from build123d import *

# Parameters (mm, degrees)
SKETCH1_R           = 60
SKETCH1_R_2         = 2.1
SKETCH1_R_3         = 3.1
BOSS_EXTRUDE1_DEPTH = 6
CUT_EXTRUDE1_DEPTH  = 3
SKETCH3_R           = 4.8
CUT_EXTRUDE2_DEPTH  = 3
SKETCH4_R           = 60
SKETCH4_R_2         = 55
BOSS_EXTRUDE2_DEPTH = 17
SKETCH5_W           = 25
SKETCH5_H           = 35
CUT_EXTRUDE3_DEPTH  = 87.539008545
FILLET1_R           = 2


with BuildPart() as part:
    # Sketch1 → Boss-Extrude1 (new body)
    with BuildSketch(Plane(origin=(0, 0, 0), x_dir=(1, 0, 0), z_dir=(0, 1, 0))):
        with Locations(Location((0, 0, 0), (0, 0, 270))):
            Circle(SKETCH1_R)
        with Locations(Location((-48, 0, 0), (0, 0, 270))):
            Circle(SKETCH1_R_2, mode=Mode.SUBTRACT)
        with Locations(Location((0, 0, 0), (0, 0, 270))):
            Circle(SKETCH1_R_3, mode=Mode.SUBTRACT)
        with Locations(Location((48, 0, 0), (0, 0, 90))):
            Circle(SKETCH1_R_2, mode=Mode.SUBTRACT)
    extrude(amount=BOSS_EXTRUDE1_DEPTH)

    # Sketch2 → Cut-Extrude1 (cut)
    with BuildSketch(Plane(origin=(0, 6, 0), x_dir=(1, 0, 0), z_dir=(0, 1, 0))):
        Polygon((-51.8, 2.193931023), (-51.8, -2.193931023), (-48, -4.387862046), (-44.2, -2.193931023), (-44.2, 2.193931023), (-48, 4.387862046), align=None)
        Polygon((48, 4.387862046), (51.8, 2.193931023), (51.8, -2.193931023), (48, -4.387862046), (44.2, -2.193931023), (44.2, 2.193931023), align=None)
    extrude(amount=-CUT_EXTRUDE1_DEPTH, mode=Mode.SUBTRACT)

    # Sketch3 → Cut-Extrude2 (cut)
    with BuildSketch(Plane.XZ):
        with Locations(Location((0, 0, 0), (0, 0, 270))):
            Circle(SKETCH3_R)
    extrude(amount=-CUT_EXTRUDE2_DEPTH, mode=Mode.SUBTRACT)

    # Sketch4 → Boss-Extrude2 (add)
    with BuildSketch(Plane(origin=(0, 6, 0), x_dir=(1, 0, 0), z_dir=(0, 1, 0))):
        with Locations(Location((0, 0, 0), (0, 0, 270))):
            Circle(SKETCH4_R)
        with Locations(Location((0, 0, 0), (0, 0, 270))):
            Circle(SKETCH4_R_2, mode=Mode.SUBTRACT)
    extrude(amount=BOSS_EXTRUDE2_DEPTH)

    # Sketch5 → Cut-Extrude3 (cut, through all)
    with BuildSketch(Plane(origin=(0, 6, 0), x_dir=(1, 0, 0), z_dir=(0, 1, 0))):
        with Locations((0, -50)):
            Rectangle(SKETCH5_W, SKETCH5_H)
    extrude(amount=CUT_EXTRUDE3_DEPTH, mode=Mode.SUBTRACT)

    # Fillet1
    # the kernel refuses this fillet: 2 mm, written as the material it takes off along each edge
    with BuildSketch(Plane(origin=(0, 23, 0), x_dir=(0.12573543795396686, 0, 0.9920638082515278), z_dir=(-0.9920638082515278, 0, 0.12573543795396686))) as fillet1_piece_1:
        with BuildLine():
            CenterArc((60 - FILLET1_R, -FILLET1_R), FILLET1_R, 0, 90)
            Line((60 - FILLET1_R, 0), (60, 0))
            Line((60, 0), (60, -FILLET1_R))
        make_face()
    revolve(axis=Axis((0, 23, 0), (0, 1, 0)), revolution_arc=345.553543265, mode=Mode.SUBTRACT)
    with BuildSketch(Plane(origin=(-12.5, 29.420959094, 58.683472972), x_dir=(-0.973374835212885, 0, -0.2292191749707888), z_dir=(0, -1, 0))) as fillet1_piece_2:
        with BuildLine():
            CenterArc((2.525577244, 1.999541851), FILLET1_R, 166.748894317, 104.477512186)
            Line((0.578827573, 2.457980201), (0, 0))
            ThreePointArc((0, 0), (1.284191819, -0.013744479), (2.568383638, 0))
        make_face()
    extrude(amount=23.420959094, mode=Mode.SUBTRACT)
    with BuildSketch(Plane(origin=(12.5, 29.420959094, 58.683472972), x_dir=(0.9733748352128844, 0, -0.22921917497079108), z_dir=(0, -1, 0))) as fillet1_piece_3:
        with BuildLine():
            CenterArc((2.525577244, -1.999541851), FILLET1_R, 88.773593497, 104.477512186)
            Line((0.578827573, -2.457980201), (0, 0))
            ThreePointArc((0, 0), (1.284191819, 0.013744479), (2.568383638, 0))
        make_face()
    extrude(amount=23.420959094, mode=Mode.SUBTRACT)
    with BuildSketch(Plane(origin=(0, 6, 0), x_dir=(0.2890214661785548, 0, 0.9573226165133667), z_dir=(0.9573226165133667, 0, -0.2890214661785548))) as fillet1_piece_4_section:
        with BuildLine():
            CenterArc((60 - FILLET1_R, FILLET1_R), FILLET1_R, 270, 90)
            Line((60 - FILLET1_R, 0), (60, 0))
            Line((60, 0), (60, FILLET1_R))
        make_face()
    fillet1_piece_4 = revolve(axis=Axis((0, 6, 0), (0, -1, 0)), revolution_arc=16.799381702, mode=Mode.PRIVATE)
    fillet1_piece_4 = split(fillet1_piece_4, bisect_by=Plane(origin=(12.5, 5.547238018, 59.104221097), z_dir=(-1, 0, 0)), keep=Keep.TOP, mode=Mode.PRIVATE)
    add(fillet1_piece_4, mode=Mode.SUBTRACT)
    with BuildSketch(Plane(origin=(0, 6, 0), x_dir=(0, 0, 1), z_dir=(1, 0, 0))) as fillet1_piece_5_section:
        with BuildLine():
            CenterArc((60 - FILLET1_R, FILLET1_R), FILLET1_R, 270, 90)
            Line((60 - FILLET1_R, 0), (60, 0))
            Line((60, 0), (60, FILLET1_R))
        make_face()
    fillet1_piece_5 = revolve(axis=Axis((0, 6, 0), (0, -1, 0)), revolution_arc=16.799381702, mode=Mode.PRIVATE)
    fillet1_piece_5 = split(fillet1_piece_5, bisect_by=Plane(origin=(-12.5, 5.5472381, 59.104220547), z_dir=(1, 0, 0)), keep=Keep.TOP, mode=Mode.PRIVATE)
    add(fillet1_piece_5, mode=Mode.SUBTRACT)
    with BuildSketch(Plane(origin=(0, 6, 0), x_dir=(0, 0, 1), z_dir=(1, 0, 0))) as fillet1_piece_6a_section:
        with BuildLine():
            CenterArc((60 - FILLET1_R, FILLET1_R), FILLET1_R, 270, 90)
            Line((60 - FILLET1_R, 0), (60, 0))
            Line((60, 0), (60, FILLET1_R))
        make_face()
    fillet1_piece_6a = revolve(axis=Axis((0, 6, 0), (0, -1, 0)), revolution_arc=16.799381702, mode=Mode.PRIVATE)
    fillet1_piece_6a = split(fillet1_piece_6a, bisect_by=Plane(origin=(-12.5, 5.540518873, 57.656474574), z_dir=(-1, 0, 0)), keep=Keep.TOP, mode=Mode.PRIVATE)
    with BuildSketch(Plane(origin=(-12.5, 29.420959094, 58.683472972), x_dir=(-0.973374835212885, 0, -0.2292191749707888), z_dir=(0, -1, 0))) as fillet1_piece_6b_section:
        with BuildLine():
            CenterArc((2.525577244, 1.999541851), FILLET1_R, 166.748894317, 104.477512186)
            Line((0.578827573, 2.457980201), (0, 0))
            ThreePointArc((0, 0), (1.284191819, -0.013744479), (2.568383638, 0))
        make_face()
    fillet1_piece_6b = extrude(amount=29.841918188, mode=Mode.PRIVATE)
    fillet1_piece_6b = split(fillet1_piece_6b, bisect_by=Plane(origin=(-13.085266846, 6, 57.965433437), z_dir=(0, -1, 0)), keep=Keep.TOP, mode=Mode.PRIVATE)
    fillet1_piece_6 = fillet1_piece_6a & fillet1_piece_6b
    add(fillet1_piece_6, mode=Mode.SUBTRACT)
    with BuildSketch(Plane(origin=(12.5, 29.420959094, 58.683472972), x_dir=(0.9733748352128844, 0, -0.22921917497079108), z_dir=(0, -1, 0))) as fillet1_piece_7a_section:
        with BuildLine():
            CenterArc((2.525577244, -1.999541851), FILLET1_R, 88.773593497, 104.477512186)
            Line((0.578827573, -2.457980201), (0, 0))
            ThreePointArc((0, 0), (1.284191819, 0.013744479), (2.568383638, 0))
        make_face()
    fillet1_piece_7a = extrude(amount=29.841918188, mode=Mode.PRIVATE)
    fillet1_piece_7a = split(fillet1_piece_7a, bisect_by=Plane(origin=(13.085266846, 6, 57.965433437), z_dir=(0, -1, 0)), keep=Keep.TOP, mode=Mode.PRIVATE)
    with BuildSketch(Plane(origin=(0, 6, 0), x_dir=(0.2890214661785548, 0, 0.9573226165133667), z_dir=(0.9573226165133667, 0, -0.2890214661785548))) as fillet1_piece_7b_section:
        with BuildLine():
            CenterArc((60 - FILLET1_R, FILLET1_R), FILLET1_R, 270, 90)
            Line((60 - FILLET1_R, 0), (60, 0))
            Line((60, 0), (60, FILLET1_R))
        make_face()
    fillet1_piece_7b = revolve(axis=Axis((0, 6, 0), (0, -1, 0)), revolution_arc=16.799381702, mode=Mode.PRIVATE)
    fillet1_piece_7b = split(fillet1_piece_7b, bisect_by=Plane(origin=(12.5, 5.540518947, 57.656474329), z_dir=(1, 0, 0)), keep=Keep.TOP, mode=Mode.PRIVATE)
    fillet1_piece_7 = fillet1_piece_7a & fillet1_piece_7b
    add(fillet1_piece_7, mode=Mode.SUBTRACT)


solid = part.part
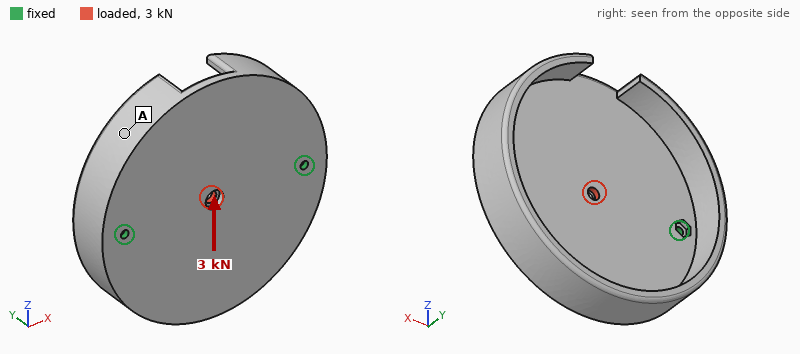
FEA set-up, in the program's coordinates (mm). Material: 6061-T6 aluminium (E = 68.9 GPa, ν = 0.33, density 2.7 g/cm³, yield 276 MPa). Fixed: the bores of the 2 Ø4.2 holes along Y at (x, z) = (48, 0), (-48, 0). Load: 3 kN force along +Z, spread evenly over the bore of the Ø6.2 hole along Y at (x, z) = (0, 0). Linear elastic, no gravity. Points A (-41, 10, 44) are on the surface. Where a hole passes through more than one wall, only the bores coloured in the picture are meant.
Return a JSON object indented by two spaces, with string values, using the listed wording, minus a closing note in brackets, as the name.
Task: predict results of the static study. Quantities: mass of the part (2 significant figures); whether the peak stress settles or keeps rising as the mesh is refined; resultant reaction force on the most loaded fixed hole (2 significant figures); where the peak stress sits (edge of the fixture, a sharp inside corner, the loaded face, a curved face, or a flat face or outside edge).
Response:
{
  "mass of the part": "260 g",
  "whether the peak stress settles or keeps rising as the mesh is refined": "keeps rising",
  "resultant reaction force on the most loaded fixed hole": "1.5 kN",
  "where the peak stress sits": "edge of the fixture"
}
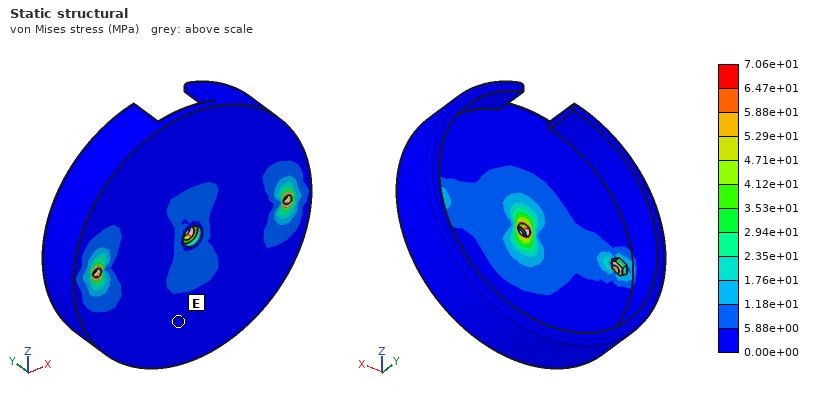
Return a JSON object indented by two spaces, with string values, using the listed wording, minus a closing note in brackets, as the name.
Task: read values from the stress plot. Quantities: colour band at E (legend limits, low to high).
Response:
{
  "colour band at E": "0.00e+00 to 5.88e+00 MPa"
}
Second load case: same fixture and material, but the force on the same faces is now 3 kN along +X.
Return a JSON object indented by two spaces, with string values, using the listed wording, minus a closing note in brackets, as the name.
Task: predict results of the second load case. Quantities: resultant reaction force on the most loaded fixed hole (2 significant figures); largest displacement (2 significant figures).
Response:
{
  "resultant reaction force on the most loaded fixed hole": "1.5 kN",
  "largest displacement": "12 µm"
}
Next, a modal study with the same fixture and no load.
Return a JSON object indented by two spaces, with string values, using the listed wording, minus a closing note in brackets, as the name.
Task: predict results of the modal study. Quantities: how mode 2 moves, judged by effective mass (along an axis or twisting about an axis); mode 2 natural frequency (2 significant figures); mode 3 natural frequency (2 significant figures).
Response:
{
  "how mode 2 moves, judged by effective mass": "along Y",
  "mode 2 natural frequency": "1600 Hz",
  "mode 3 natural frequency": "2500 Hz"
}
